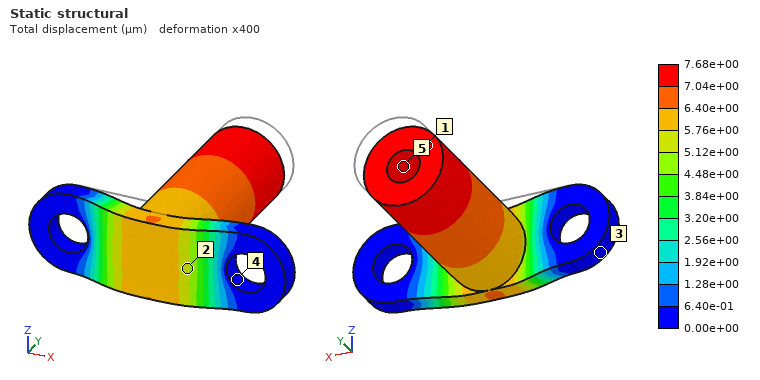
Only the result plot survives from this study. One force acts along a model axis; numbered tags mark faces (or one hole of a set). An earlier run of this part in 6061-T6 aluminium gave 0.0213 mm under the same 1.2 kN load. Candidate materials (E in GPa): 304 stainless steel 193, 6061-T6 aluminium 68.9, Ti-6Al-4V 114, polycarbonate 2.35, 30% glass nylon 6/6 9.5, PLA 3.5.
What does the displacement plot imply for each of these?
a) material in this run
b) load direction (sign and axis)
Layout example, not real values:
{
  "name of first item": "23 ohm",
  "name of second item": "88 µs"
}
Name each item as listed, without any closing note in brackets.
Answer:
{
  "material in this run": "304 stainless steel",
  "load direction": "-Y"
}
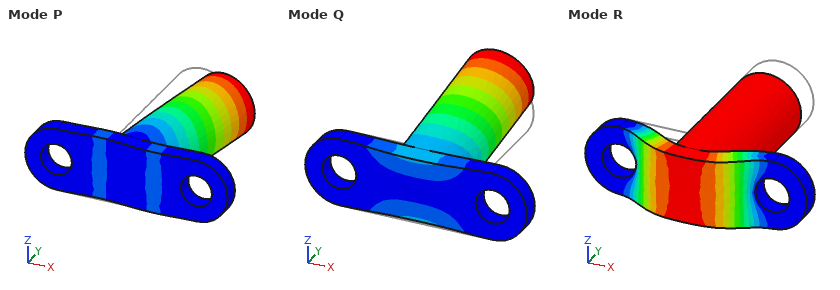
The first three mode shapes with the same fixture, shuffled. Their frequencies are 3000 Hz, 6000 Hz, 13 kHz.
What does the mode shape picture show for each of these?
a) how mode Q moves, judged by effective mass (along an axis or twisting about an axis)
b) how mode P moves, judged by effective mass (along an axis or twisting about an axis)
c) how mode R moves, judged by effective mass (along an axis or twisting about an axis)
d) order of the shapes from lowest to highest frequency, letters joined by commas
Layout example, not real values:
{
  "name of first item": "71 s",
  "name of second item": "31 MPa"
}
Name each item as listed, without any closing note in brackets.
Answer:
{
  "how mode Q moves, judged by effective mass": "along Z",
  "how mode P moves, judged by effective mass": "along X",
  "how mode R moves, judged by effective mass": "along Y",
  "order of the shapes from lowest to highest frequency, letters joined by commas": "Q, P, R"
}
